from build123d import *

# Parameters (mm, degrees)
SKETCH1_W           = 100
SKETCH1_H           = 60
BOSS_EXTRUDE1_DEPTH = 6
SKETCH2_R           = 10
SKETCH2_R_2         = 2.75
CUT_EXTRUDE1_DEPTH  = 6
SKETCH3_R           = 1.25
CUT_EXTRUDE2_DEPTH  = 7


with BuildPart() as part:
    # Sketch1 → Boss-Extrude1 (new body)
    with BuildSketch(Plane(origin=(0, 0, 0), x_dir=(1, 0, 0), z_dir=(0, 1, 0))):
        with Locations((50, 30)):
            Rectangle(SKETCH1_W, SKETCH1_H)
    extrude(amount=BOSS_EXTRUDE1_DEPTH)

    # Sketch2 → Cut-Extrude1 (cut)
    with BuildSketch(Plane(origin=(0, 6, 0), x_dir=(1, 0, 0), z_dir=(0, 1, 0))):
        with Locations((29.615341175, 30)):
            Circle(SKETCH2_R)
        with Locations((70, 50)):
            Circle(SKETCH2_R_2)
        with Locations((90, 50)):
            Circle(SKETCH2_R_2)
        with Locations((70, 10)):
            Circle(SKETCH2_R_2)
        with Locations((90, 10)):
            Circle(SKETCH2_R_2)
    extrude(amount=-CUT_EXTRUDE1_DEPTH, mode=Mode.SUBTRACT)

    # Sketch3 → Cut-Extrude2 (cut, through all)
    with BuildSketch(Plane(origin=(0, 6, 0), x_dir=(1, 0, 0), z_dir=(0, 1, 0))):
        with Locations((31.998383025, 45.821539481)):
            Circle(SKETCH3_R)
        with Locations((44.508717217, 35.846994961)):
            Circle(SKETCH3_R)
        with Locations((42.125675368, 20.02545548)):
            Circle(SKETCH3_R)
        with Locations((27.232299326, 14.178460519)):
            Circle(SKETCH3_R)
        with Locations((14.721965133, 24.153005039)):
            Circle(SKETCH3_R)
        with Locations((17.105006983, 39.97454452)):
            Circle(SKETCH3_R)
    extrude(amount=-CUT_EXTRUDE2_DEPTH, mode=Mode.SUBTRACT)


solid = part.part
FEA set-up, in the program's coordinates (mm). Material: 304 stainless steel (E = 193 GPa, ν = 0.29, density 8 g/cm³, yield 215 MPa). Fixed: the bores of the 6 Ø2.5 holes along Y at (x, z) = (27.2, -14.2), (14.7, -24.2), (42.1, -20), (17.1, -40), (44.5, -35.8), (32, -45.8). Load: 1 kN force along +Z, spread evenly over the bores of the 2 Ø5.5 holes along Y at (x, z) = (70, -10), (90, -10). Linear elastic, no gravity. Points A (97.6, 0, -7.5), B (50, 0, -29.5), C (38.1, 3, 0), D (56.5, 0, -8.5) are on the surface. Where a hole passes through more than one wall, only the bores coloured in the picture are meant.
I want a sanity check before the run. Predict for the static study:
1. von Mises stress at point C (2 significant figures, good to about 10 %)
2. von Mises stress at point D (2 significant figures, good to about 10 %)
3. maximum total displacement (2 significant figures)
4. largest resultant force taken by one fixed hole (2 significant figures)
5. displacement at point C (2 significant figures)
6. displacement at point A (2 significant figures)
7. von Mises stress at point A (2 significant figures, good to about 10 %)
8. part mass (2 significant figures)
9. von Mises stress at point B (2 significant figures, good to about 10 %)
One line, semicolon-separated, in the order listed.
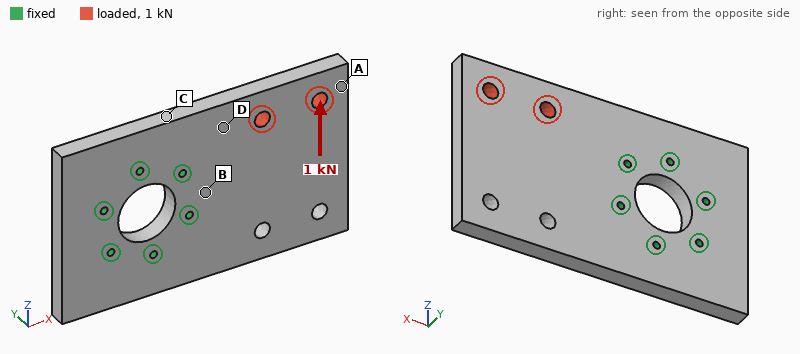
9.0 MPa; 5.6 MPa; 6.1 µm; 820 N; 1.1 µm; 5.8 µm; 1.7 MPa; 270 g; 11 MPa
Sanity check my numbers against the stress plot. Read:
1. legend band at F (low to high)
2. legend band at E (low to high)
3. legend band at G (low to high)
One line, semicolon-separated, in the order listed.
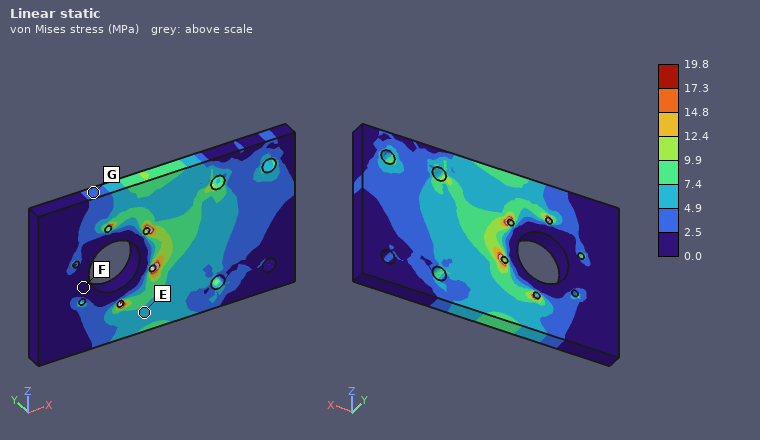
0.0 to 2.5 MPa; 4.9 to 7.4 MPa; 2.5 to 4.9 MPa
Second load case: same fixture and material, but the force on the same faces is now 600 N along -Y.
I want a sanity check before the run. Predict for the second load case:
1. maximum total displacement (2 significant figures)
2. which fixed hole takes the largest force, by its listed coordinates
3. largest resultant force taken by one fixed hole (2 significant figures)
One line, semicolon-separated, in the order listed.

0.15 mm; (42.1, -20); 870 N
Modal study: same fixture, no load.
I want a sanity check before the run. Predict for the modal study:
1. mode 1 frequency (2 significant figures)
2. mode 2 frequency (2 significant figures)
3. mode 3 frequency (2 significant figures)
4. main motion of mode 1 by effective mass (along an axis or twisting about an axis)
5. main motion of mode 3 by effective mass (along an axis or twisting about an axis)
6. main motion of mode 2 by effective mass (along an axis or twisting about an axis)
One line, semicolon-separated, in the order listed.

1400 Hz; 2800 Hz; 6900 Hz; along Y; along Z; twisting about X
